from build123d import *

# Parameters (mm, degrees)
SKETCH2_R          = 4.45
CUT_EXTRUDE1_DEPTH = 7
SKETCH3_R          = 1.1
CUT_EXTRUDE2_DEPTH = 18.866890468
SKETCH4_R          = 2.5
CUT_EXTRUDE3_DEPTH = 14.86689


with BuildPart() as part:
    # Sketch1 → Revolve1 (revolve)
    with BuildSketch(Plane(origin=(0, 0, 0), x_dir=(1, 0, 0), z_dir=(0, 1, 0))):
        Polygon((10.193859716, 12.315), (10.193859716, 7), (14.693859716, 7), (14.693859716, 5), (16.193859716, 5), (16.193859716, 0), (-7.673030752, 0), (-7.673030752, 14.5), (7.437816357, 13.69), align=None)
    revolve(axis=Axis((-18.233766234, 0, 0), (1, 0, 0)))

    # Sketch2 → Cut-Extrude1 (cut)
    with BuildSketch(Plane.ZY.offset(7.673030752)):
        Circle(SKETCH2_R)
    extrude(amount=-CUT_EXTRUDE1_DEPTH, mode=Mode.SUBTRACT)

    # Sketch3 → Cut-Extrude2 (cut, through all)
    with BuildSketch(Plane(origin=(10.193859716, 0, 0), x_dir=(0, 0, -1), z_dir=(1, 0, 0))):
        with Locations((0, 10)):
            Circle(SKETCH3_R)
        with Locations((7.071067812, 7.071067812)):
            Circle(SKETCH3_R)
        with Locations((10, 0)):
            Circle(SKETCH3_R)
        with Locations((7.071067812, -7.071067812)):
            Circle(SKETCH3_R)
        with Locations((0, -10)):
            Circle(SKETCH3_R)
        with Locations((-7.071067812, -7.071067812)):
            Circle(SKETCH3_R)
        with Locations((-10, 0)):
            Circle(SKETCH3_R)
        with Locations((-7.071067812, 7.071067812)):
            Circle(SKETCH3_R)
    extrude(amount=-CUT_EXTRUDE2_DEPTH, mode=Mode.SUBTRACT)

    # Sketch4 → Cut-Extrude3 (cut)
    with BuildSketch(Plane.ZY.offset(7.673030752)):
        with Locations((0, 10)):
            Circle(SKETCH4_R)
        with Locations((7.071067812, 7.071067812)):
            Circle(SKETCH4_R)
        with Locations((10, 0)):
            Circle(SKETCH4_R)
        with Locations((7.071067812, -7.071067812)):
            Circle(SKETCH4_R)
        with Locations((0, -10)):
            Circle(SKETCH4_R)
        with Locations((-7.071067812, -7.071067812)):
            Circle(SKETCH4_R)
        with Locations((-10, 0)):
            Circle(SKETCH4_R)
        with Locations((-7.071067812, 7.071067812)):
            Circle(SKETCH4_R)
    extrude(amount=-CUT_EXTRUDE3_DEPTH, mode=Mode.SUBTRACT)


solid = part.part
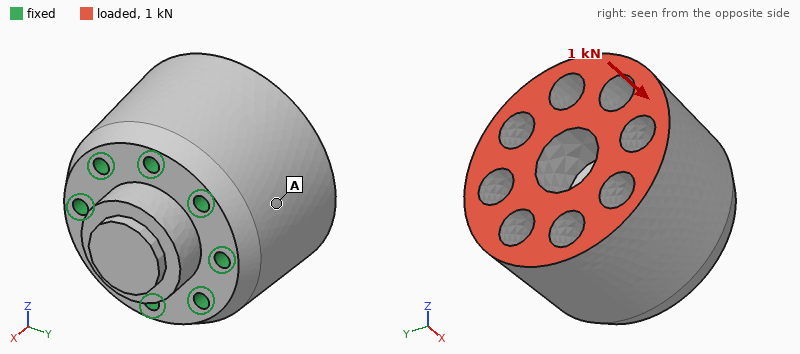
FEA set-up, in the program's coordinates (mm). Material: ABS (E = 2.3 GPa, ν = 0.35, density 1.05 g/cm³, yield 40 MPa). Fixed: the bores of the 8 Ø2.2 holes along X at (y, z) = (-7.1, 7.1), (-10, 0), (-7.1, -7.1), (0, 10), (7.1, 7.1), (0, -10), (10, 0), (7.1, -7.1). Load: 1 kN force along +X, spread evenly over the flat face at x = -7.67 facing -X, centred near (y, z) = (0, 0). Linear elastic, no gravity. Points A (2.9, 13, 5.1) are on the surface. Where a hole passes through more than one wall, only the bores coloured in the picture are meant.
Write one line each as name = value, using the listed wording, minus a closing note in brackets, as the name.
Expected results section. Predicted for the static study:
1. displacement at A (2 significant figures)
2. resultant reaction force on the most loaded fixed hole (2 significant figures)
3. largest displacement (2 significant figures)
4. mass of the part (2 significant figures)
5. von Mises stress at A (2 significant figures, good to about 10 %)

displacement at A = 19 µm
resultant reaction force on the most loaded fixed hole = 130 N
largest displacement = 31 µm
mass of the part = 9.3 g
von Mises stress at A = 2.2 MPa
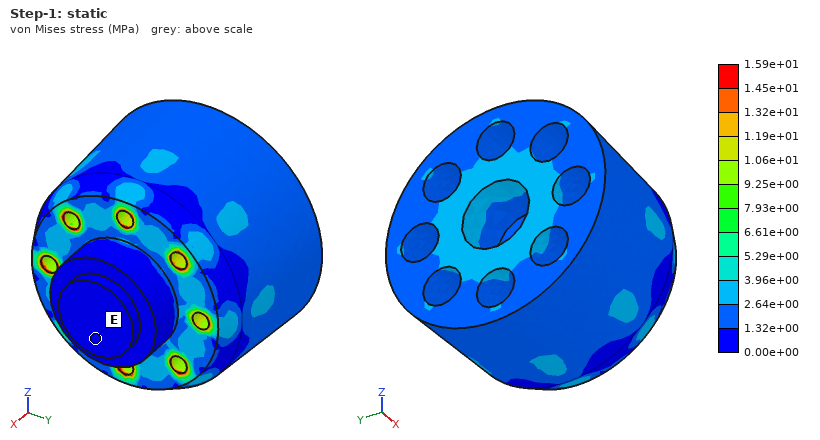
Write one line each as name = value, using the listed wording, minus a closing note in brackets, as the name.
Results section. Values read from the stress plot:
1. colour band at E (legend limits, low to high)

colour band at E = 0.00e+00 to 1.32e+00 MPa
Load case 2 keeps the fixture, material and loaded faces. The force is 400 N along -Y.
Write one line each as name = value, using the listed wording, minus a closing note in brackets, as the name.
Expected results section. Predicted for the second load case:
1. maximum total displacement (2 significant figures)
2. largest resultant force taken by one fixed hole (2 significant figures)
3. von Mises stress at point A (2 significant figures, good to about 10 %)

maximum total displacement = 82 µm
largest resultant force taken by one fixed hole = 160 N
von Mises stress at point A = 2.3 MPa
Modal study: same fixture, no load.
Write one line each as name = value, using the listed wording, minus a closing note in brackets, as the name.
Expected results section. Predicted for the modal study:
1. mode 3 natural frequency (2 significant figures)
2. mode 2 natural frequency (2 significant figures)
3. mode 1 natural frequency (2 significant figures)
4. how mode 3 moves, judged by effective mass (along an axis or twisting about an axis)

mode 3 natural frequency = 11 kHz
mode 2 natural frequency = 7300 Hz
mode 1 natural frequency = 7300 Hz
how mode 3 moves, judged by effective mass = twisting about X
